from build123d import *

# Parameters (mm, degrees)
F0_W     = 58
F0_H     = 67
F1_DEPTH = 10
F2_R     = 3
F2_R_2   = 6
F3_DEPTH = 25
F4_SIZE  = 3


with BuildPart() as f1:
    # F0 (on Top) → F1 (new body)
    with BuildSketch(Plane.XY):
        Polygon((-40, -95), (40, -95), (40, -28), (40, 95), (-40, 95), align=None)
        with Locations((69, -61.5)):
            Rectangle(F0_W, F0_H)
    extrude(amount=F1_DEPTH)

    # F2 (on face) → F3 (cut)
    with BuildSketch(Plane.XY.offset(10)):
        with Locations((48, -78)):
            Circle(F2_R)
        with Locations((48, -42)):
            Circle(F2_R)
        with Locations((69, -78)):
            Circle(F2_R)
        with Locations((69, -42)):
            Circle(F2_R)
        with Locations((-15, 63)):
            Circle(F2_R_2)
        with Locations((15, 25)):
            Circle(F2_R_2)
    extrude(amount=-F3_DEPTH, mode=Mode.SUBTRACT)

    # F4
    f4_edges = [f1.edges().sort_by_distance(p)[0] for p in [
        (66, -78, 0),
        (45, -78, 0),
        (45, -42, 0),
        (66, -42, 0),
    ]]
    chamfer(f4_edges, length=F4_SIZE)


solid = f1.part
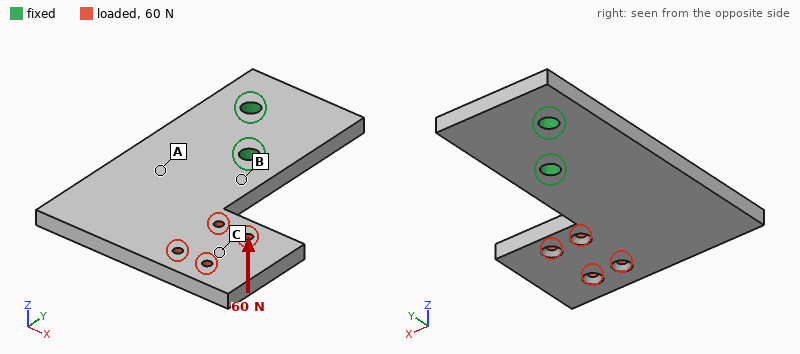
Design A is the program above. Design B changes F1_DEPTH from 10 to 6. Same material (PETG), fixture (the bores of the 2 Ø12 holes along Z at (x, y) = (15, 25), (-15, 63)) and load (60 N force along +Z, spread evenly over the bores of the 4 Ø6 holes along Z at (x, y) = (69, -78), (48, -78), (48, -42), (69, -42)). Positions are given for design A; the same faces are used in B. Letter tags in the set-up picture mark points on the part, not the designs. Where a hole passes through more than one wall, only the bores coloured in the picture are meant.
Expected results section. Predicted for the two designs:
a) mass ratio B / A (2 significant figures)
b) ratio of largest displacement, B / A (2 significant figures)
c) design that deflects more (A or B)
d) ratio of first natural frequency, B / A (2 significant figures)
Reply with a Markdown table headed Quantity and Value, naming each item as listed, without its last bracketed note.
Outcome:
| Quantity | Value |
|---|---|
| mass ratio B / A | 0.60 |
| ratio of largest displacement, B / A | 4.5 |
| design that deflects more | B |
| ratio of first natural frequency, B / A | 0.61 |
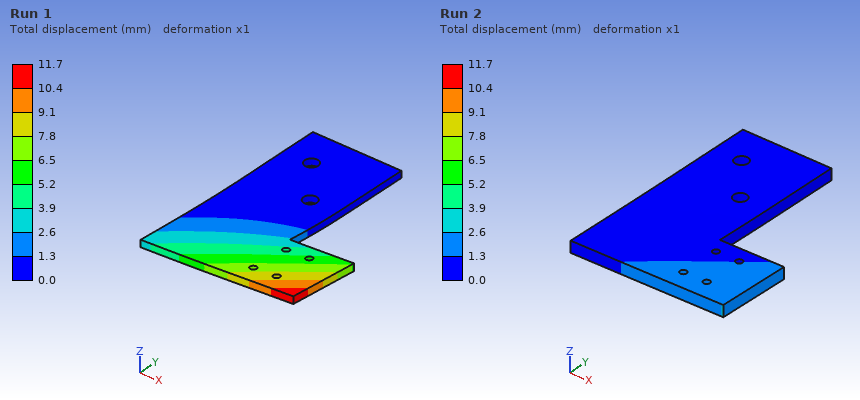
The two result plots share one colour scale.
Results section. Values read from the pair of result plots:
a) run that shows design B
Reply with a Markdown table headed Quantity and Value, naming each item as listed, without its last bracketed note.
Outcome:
| Quantity | Value |
|---|---|
| run that shows design B | Run 1 |
